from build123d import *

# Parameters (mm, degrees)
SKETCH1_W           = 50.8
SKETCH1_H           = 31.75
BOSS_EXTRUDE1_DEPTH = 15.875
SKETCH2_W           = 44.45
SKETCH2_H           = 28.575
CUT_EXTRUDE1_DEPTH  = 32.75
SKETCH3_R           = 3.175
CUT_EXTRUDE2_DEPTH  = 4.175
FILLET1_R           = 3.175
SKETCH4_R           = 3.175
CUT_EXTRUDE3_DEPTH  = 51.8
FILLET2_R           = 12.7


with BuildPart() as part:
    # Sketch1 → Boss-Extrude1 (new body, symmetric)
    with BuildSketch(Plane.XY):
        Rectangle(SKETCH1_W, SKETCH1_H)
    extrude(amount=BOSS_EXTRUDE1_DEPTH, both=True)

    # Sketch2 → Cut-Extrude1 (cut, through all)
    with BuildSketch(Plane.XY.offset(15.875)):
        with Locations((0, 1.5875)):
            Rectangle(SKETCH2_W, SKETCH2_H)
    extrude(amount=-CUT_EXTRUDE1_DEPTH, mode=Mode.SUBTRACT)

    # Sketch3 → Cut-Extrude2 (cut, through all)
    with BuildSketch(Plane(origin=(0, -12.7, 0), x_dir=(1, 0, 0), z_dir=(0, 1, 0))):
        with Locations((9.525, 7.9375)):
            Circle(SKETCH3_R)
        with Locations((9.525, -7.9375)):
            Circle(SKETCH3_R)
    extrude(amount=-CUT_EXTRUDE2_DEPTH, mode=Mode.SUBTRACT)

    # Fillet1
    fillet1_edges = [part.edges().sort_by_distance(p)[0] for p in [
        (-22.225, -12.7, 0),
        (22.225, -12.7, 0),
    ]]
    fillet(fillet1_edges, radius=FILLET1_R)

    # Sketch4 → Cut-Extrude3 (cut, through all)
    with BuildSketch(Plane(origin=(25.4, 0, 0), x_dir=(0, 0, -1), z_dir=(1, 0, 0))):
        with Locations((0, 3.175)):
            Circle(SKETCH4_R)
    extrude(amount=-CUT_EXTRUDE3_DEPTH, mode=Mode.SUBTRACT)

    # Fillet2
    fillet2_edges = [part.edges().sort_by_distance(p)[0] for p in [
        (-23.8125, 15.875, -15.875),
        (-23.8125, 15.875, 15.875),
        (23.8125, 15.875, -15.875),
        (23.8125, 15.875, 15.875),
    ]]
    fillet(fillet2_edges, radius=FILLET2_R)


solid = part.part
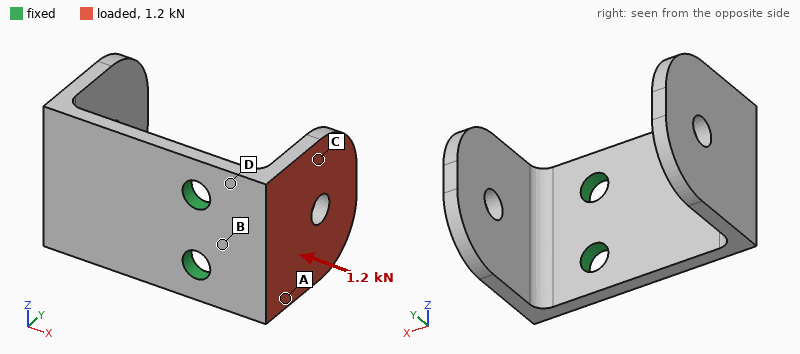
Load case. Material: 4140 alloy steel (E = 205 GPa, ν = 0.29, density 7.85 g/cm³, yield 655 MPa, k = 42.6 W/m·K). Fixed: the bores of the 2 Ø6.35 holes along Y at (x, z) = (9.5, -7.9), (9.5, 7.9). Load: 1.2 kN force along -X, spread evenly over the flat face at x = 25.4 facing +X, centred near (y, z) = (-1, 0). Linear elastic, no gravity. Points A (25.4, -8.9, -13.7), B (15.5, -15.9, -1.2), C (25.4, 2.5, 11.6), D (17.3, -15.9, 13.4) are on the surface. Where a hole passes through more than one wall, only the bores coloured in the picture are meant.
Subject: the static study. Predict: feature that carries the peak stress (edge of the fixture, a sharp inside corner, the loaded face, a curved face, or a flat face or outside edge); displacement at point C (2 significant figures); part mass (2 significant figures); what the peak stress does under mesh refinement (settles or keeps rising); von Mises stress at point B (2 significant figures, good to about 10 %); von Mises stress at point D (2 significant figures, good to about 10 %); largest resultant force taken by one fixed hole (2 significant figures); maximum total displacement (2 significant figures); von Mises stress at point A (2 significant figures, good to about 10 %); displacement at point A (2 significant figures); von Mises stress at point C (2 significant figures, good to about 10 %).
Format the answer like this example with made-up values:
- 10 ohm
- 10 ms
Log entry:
- edge of the fixture
- 0.22 mm
- 80 g
- keeps rising
- 230 MPa
- 270 MPa
- 620 N
- 0.42 mm
- 190 MPa
- 0.096 mm
- 61 MPa
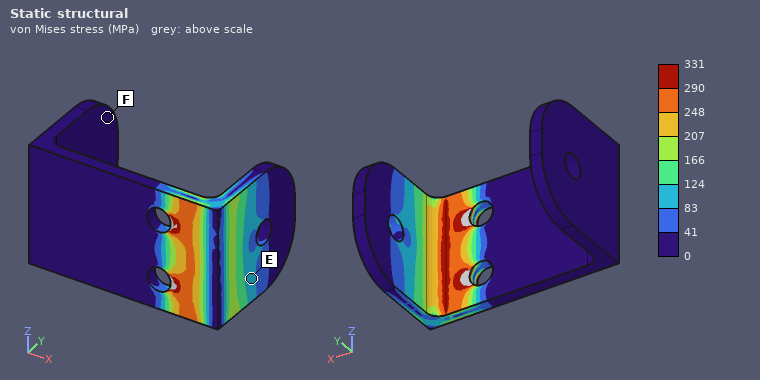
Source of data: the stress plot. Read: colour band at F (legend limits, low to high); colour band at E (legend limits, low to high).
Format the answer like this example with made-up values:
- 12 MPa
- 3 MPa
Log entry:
- 0 to 41 MPa
- 83 to 124 MPa
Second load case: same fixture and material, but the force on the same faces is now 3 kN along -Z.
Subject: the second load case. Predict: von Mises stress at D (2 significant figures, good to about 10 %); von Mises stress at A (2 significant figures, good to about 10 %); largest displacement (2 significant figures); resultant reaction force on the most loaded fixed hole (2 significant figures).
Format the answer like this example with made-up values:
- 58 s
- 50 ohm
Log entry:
- 140 MPa
- 120 MPa
- 0.17 mm
- 3.2 kN
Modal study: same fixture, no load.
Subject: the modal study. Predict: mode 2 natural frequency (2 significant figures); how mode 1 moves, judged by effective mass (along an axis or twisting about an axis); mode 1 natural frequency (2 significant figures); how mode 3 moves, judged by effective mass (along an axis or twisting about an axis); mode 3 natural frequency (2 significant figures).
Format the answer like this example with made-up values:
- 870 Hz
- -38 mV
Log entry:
- 2000 Hz
- along Y
- 1000 Hz
- along X
- 2200 Hz
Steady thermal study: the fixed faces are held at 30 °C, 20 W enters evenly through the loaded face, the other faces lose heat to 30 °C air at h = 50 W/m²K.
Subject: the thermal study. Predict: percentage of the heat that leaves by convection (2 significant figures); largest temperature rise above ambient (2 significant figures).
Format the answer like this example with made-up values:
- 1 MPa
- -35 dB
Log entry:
- 25 %
- 86 K
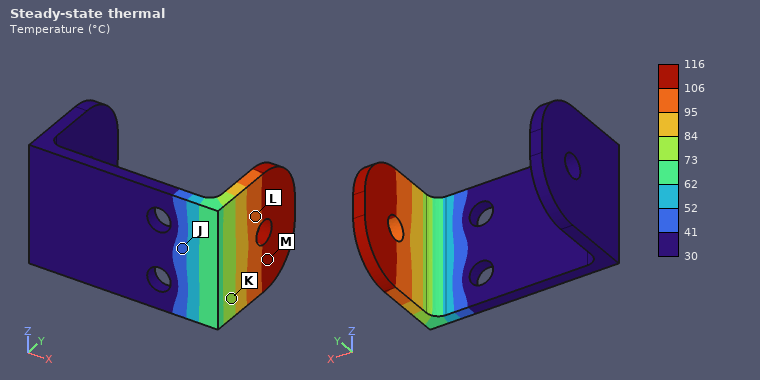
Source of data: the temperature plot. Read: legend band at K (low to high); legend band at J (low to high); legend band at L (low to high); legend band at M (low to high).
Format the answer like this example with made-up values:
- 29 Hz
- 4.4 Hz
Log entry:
- 73 to 84 °C
- 41 to 52 °C
- 95 to 106 °C
- 106 to 116 °C
